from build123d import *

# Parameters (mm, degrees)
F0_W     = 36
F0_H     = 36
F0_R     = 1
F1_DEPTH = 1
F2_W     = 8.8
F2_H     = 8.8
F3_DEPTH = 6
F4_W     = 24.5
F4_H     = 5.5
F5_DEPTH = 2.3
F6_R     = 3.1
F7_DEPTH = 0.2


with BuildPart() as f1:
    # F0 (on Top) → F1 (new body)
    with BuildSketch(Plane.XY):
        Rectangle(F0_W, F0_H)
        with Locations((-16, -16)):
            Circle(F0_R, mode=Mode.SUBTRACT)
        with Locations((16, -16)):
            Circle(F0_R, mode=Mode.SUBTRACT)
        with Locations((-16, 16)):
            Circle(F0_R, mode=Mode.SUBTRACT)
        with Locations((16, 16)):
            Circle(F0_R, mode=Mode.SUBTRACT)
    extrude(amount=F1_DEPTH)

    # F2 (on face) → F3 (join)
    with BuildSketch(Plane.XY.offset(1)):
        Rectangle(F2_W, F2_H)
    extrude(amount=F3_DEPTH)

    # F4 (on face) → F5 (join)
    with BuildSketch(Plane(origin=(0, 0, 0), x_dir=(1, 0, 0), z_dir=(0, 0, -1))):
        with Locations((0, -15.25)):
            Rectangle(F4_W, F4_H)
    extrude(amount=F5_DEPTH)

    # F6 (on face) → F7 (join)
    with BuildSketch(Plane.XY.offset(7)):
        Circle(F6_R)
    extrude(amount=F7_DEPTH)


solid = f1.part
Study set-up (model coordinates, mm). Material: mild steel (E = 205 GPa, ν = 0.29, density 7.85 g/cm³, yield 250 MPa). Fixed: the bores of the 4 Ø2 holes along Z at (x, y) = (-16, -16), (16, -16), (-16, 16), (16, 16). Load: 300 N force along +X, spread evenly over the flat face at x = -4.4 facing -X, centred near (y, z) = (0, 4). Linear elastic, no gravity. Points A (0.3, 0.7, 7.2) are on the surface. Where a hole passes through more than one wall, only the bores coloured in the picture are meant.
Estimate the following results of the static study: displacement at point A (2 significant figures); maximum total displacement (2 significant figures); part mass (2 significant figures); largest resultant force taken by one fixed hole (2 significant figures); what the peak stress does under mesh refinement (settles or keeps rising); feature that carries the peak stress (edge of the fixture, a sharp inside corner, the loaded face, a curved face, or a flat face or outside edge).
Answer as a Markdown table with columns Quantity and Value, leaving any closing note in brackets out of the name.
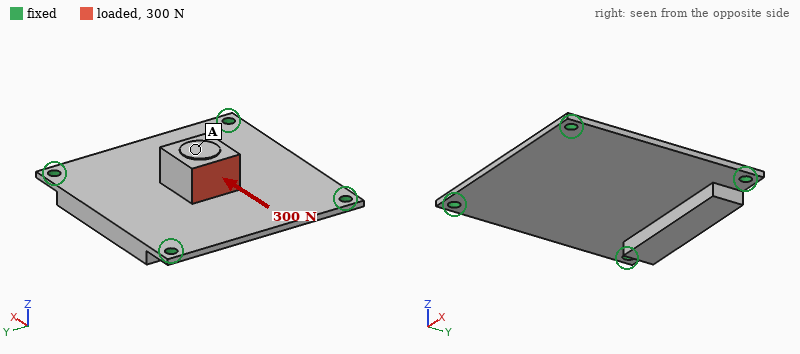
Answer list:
| Quantity | Value |
|---|---|
| displacement at point A | 22 µm |
| maximum total displacement | 25 µm |
| part mass | 16 g |
| largest resultant force taken by one fixed hole | 92 N |
| what the peak stress does under mesh refinement | keeps rising |
| feature that carries the peak stress | edge of the fixture |
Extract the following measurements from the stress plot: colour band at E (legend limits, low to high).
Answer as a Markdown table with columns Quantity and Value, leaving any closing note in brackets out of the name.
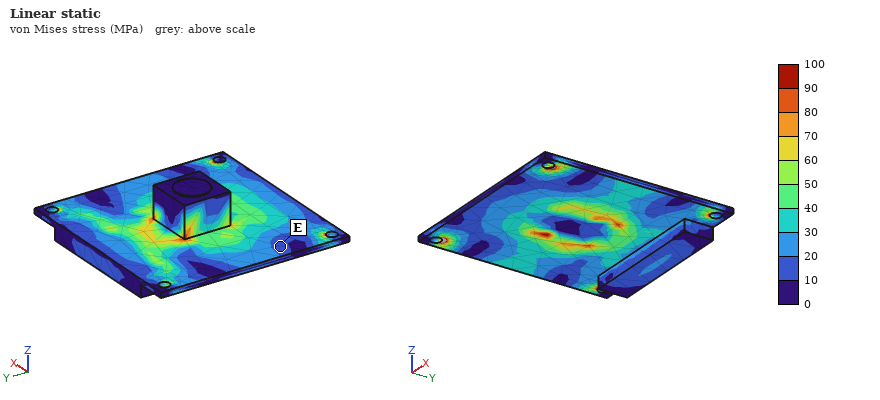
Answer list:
| Quantity | Value |
|---|---|
| colour band at E | 10 to 20 MPa |
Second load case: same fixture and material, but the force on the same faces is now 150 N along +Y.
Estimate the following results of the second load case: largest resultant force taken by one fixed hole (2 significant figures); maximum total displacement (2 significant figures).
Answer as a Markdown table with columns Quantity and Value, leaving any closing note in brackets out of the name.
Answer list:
| Quantity | Value |
|---|---|
| largest resultant force taken by one fixed hole | 46 N |
| maximum total displacement | 15 µm |
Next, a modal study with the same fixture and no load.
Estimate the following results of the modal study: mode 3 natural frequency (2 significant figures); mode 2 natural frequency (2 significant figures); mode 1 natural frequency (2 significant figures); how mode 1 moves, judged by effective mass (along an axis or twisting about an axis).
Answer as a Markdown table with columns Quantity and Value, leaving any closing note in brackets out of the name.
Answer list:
| Quantity | Value |
|---|---|
| mode 3 natural frequency | 6200 Hz |
| mode 2 natural frequency | 5900 Hz |
| mode 1 natural frequency | 3000 Hz |
| how mode 1 moves, judged by effective mass | along Z |
